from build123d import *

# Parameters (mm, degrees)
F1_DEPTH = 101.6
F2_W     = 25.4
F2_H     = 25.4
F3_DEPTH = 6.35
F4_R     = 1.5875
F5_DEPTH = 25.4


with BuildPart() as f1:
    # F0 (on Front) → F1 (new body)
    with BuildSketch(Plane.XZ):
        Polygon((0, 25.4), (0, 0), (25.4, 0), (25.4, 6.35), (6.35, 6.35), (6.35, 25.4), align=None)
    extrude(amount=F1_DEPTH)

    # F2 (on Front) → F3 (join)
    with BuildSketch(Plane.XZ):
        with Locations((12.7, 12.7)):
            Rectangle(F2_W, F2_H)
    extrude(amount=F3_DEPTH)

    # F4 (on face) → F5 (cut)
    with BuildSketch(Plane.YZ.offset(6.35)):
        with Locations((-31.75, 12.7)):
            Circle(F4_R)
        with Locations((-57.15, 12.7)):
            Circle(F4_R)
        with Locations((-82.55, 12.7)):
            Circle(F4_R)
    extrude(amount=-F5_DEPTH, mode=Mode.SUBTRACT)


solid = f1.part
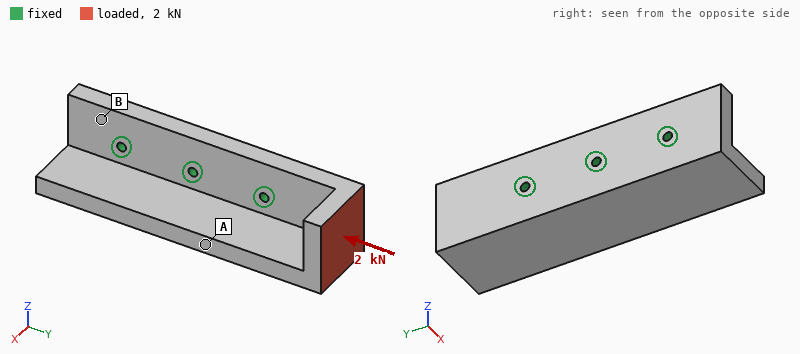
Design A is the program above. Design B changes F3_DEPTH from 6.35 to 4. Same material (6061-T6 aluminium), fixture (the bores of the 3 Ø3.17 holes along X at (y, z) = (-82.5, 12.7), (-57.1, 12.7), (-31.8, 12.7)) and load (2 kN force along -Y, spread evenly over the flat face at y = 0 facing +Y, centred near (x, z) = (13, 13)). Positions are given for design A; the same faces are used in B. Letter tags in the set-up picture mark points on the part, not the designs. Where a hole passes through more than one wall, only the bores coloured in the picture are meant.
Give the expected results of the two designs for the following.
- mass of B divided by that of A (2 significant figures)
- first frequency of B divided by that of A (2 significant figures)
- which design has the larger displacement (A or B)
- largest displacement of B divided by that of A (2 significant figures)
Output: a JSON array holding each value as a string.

["0.97", "1.0", "B", "1.7"]
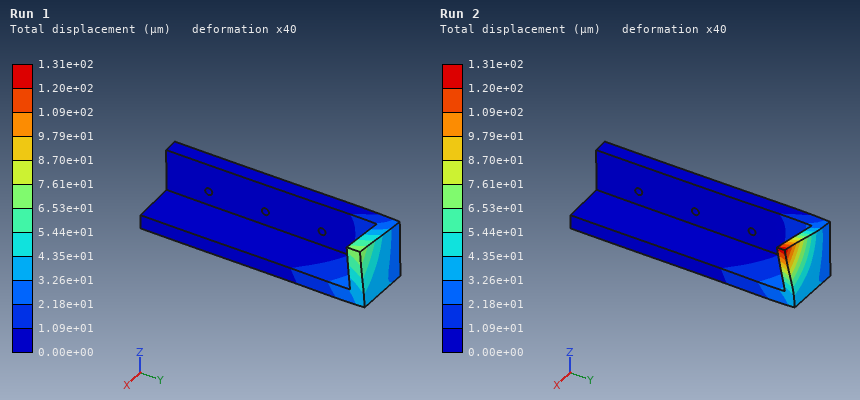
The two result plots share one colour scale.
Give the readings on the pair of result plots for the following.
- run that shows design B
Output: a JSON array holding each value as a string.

["Run 2"]
